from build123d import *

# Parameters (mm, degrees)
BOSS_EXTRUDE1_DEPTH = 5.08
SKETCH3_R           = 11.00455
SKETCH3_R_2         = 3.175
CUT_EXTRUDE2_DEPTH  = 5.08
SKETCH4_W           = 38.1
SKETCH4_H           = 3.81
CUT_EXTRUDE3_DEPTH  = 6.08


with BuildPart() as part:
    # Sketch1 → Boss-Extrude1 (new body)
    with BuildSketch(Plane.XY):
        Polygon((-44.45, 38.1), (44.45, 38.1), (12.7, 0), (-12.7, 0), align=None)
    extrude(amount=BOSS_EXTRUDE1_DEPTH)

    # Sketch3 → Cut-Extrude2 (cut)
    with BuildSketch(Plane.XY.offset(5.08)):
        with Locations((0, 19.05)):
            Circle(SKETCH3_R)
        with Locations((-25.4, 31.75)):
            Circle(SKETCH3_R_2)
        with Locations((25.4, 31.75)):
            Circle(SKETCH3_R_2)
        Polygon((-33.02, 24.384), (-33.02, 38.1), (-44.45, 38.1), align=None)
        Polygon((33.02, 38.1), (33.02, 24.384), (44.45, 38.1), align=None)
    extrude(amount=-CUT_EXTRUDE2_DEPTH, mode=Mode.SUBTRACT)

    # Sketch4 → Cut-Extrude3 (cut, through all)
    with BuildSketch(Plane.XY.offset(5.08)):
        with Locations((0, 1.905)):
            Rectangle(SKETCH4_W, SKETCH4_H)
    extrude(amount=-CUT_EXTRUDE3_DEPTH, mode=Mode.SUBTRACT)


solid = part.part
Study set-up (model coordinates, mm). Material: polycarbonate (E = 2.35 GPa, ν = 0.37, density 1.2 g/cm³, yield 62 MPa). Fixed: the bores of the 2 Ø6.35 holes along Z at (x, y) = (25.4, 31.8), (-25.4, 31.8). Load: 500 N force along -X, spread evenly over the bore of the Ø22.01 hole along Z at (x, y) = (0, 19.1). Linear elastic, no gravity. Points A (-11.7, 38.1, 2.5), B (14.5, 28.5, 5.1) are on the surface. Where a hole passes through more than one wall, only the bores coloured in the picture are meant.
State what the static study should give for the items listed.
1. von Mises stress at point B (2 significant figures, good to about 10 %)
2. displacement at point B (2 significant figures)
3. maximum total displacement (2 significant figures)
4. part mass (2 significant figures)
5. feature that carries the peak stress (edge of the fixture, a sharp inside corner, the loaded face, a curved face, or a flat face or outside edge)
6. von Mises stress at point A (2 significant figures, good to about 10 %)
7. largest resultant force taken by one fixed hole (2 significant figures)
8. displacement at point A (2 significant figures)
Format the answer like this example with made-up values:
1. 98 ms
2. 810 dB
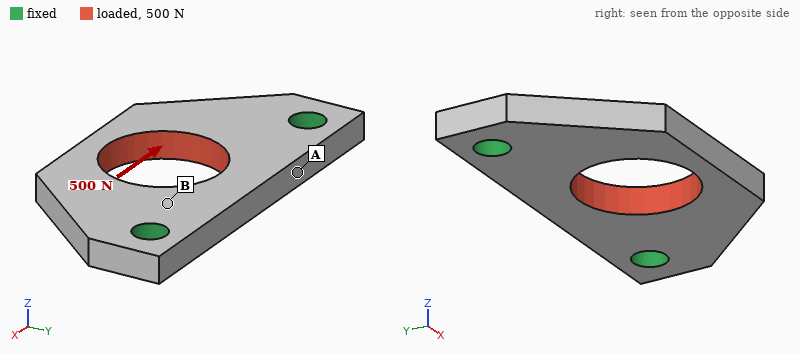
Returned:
1. 1.9 MPa
2. 0.022 mm
3. 0.11 mm
4. 8.9 g
5. edge of the fixture
6. 4.1 MPa
7. 260 N
8. 0.017 mm
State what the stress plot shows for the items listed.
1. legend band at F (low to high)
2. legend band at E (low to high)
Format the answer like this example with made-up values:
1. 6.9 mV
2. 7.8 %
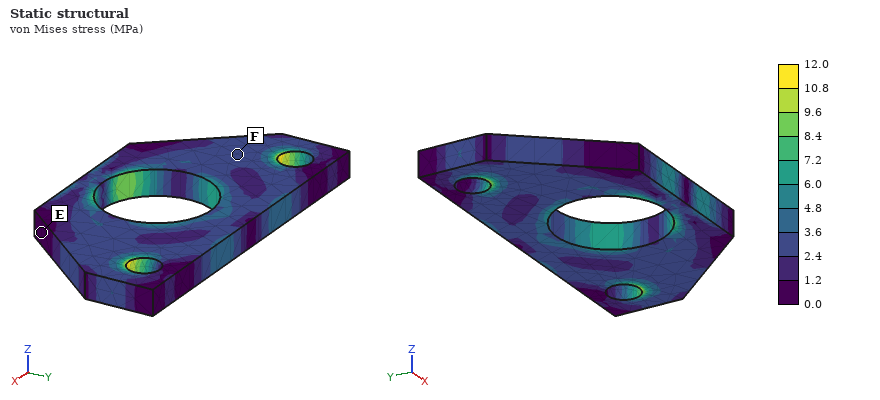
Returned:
1. 2.4 to 3.6 MPa
2. 0.0 to 1.2 MPa
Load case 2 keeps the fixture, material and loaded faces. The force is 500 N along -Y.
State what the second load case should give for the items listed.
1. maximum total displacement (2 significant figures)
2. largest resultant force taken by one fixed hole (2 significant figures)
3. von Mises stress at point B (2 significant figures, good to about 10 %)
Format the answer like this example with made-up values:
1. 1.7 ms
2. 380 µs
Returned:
1. 79 µm
2. 260 N
3. 2.7 MPa
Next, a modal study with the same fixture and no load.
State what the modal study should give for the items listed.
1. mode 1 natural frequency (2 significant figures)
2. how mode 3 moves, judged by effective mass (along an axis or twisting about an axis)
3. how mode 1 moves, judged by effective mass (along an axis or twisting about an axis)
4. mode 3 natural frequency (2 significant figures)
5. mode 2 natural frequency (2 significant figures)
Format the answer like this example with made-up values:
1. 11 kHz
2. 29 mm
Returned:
1. 1400 Hz
2. along Z
3. along Z
4. 3400 Hz
5. 2900 Hz
